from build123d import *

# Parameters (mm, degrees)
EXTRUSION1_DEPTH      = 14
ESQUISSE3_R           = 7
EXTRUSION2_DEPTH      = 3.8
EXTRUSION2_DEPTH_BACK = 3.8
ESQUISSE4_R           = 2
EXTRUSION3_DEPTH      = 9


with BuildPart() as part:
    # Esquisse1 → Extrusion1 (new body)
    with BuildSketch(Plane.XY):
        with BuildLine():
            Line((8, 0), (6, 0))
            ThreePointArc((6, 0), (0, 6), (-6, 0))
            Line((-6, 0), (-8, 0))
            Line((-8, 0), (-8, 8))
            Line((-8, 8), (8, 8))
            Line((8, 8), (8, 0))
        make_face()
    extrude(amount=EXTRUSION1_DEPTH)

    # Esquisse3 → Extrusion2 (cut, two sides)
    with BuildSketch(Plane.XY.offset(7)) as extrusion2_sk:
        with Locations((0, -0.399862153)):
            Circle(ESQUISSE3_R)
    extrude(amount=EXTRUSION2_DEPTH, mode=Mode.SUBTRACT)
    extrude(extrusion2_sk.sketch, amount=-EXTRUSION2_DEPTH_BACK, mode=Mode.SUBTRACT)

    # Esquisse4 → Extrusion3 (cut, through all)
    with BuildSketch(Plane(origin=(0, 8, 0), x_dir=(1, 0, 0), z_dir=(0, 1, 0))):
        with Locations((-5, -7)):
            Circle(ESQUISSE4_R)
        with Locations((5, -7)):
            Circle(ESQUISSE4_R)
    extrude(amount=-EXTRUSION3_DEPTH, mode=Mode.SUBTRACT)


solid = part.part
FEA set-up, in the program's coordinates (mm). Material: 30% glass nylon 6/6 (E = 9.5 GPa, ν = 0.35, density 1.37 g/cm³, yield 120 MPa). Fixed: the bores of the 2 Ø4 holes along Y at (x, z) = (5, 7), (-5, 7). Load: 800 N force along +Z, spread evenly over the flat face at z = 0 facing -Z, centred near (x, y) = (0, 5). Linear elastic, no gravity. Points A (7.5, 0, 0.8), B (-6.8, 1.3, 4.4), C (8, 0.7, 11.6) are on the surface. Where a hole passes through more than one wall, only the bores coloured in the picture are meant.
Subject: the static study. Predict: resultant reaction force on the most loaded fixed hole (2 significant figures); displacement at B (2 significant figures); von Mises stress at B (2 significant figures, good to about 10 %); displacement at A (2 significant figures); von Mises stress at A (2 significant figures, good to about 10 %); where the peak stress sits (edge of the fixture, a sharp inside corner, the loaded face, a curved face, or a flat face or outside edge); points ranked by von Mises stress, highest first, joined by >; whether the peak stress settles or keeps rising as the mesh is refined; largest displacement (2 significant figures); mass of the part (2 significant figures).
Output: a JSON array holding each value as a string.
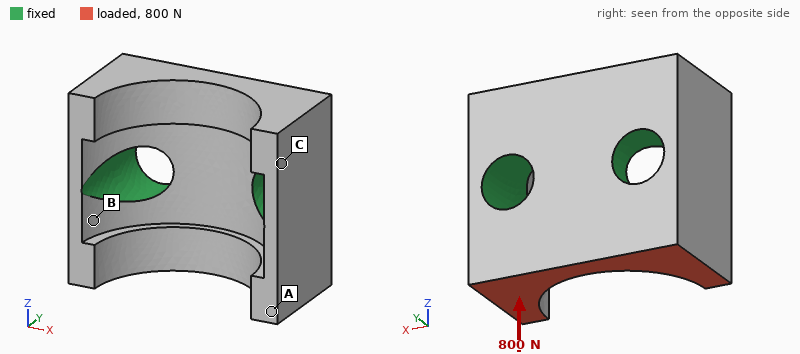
["400 N", "6.0 µm", "24 MPa", "14 µm", "12 MPa", "edge of the fixture", "B > A > C", "keeps rising", "18 µm", "1.1 g"]
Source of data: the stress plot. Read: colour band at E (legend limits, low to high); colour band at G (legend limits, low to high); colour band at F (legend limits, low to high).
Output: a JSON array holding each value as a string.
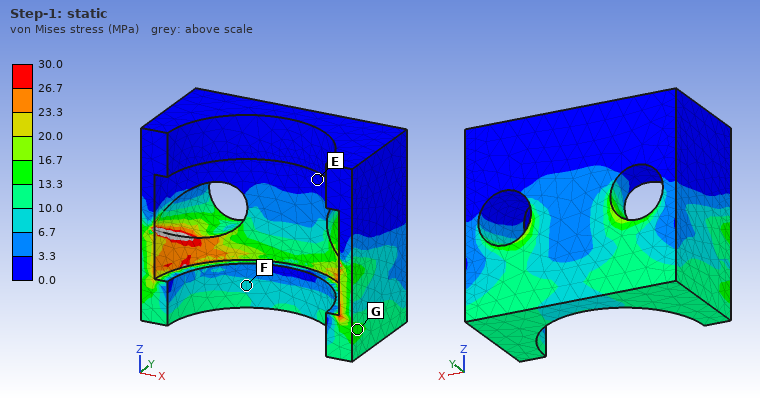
["0.0 to 3.3 MPa", "13.3 to 16.7 MPa", "6.7 to 10.0 MPa"]
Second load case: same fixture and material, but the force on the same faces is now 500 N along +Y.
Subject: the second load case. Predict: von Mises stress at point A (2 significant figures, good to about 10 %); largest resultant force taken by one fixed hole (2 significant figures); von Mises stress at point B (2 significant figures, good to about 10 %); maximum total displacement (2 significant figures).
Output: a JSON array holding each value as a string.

["11 MPa", "260 N", "46 MPa", "62 µm"]
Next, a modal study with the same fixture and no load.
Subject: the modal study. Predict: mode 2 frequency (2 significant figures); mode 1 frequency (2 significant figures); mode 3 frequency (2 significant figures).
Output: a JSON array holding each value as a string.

["35 kHz", "34 kHz", "35 kHz"]
